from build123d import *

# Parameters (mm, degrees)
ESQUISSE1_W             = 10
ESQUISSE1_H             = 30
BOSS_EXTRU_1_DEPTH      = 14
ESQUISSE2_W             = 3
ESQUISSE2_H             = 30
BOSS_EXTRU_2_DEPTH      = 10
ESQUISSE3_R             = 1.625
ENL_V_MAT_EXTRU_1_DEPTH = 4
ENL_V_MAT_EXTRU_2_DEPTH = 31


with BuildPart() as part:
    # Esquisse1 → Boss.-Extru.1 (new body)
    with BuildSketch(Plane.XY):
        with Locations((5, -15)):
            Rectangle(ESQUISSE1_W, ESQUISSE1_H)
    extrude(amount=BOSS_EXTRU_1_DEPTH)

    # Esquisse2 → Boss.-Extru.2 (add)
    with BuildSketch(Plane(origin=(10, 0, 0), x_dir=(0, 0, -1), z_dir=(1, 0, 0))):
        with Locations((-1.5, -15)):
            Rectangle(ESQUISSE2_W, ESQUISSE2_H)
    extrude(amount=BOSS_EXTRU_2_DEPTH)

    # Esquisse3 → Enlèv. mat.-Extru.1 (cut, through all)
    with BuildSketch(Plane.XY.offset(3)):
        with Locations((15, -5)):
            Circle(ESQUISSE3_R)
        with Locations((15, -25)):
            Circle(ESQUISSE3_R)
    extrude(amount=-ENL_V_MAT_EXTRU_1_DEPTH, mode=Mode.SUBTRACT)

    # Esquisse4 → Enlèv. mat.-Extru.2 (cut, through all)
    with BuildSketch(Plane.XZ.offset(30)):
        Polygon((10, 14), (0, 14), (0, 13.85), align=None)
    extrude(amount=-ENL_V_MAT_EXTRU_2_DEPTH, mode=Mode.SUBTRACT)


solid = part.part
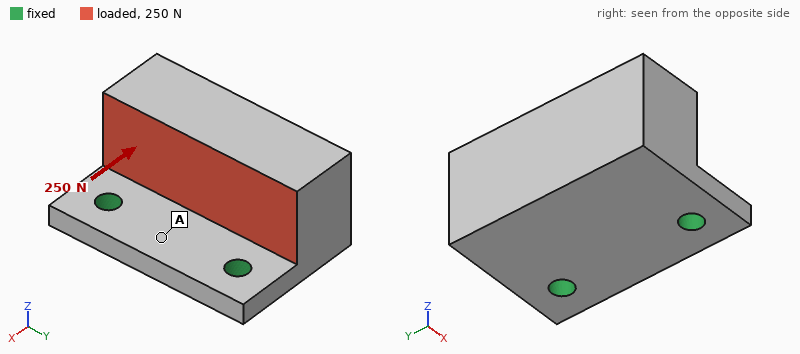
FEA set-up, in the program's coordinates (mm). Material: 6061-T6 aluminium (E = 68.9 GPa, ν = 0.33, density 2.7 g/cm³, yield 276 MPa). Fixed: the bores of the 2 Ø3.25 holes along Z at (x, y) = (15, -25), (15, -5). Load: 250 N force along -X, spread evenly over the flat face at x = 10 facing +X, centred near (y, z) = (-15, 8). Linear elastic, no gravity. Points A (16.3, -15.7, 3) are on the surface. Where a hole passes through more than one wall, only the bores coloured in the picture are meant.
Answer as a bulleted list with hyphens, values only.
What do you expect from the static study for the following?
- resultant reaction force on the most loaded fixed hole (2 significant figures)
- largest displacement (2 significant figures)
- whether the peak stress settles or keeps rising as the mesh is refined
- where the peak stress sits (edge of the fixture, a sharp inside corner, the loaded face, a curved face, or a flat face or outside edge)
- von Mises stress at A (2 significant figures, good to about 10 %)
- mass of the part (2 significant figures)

- 130 N
- 41 µm
- keeps rising
- edge of the fixture
- 9.8 MPa
- 14 g
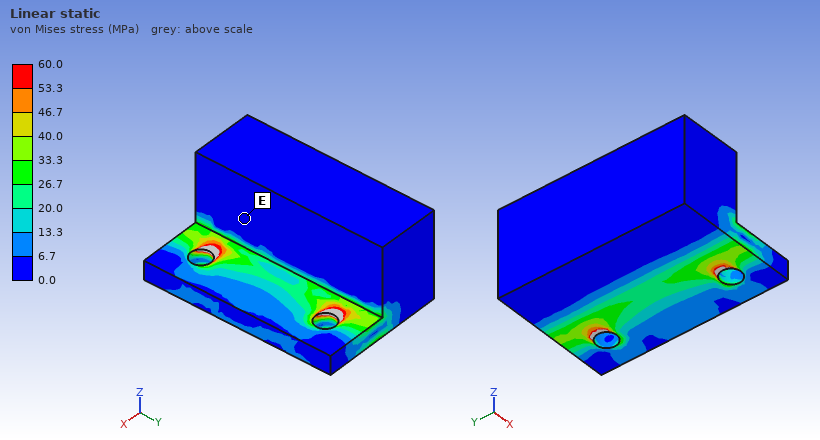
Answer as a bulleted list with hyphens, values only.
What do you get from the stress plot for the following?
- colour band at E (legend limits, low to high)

- 0.0 to 6.7 MPa
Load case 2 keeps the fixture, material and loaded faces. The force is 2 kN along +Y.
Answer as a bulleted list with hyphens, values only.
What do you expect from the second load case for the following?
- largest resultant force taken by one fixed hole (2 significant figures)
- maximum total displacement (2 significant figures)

- 1.3 kN
- 40 µm
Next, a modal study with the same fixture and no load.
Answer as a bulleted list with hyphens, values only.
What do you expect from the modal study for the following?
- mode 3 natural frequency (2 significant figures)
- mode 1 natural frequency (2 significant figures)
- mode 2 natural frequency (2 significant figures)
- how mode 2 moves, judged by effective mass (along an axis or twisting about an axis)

- 20 kHz
- 4000 Hz
- 13 kHz
- along Y
